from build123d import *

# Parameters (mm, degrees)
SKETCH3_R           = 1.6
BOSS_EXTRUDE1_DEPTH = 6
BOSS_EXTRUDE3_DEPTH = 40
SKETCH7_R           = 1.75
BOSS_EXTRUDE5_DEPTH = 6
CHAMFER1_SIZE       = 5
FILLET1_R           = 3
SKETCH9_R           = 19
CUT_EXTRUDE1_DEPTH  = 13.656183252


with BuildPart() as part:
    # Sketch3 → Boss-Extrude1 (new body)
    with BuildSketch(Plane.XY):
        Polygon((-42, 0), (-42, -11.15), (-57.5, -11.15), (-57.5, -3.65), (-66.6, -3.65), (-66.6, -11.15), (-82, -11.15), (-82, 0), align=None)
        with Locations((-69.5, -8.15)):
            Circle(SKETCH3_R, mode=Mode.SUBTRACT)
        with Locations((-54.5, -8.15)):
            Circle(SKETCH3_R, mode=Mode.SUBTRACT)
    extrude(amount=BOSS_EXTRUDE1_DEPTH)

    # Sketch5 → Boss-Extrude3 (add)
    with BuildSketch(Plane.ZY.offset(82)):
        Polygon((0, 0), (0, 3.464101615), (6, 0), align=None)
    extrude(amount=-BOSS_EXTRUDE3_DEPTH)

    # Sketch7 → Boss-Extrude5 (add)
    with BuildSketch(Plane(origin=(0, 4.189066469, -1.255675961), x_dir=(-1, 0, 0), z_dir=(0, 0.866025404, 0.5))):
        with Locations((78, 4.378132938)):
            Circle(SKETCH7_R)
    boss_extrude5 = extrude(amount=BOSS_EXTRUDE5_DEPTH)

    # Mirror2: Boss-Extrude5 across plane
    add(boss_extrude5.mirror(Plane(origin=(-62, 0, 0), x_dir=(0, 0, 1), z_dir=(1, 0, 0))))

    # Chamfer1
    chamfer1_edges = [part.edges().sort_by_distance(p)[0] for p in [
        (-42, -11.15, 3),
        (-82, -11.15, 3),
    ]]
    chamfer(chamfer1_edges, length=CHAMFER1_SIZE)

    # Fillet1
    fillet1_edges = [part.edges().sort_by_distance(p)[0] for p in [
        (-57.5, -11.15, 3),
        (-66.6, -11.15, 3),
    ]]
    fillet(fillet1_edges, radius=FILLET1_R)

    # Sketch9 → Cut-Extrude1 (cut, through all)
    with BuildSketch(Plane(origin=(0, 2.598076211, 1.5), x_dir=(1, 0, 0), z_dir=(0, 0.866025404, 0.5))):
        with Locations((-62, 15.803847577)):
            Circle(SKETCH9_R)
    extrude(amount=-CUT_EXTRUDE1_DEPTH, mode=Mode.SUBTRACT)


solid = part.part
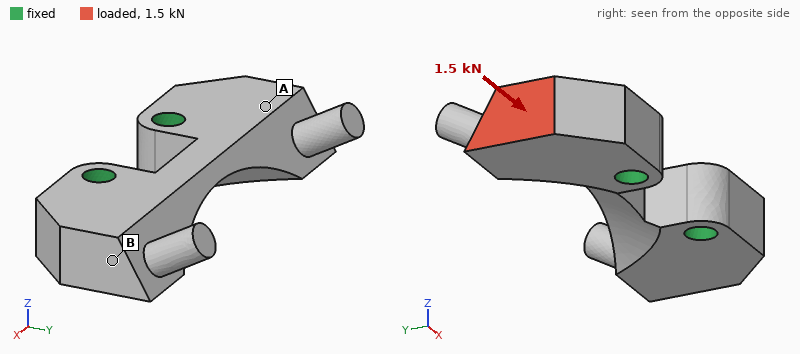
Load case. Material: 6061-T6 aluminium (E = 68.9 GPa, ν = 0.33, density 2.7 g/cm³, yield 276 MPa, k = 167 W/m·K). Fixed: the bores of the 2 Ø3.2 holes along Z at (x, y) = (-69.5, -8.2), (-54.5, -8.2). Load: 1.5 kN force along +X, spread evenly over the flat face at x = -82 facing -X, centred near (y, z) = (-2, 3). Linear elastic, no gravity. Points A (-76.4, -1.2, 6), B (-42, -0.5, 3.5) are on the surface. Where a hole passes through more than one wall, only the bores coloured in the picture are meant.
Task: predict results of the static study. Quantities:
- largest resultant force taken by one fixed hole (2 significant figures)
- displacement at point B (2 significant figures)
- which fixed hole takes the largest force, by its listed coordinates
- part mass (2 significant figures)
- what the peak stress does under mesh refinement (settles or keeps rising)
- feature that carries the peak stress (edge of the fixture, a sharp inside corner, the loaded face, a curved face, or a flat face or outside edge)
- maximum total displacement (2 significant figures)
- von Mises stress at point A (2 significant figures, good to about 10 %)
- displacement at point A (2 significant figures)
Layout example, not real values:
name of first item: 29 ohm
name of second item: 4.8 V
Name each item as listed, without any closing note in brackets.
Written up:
largest resultant force taken by one fixed hole: 1.1 kN
displacement at point B: 6.9 µm
which fixed hole takes the largest force, by its listed coordinates: (-69.5, -8.2)
part mass: 6.1 g
what the peak stress does under mesh refinement: keeps rising
feature that carries the peak stress: edge of the fixture
maximum total displacement: 37 µm
von Mises stress at point A: 37 MPa
displacement at point A: 18 µm
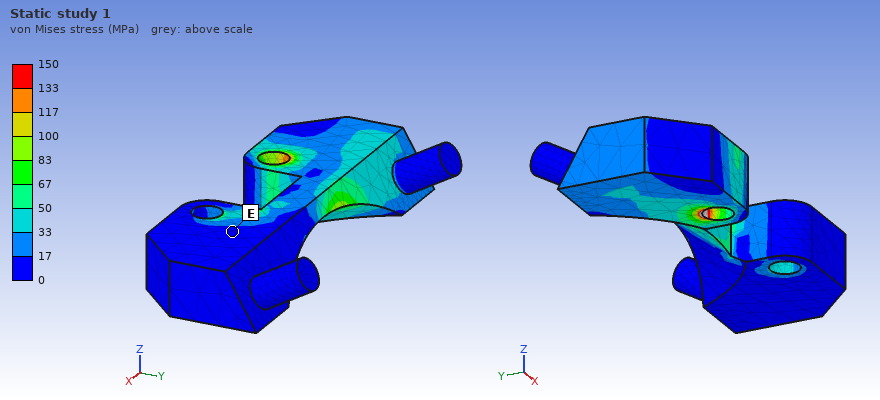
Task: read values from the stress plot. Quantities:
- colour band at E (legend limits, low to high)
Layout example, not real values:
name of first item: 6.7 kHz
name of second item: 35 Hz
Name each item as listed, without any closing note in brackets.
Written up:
colour band at E: 0 to 17 MPa
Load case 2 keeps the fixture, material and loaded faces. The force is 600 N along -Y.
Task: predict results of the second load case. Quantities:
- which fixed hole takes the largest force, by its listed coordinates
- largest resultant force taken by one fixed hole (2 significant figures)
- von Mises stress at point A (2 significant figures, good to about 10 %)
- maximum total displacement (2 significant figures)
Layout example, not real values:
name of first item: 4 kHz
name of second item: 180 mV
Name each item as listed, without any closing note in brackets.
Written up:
which fixed hole takes the largest force, by its listed coordinates: (-69.5, -8.2)
largest resultant force taken by one fixed hole: 760 N
von Mises stress at point A: 19 MPa
maximum total displacement: 33 µm
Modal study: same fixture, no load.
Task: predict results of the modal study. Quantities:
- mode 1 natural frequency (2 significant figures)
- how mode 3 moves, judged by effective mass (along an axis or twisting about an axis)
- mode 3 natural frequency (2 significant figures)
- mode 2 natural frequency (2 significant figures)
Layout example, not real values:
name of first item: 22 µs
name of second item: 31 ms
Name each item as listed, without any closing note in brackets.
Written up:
mode 1 natural frequency: 20 kHz
how mode 3 moves, judged by effective mass: along X
mode 3 natural frequency: 21 kHz
mode 2 natural frequency: 20 kHz
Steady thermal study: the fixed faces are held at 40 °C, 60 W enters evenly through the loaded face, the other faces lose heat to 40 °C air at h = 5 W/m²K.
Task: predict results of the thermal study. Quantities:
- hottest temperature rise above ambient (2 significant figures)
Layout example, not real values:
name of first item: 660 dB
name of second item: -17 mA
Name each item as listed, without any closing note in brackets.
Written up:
hottest temperature rise above ambient: 84 K
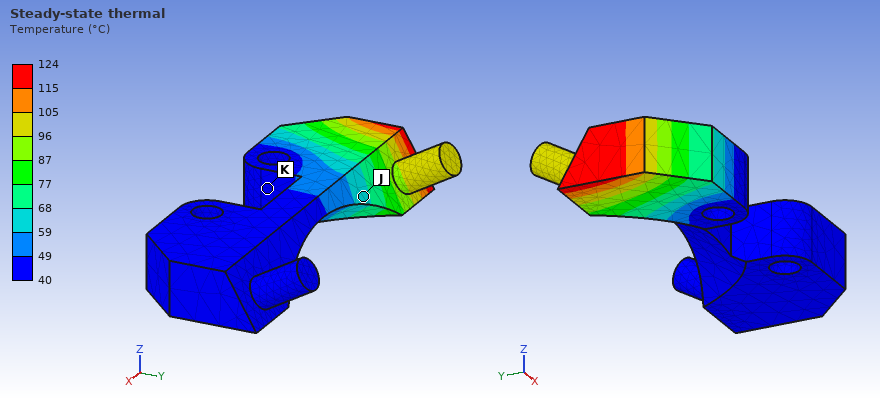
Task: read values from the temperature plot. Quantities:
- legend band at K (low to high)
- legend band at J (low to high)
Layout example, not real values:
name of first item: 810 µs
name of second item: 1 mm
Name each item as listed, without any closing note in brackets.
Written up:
legend band at K: 40 to 49 °C
legend band at J: 59 to 68 °C
